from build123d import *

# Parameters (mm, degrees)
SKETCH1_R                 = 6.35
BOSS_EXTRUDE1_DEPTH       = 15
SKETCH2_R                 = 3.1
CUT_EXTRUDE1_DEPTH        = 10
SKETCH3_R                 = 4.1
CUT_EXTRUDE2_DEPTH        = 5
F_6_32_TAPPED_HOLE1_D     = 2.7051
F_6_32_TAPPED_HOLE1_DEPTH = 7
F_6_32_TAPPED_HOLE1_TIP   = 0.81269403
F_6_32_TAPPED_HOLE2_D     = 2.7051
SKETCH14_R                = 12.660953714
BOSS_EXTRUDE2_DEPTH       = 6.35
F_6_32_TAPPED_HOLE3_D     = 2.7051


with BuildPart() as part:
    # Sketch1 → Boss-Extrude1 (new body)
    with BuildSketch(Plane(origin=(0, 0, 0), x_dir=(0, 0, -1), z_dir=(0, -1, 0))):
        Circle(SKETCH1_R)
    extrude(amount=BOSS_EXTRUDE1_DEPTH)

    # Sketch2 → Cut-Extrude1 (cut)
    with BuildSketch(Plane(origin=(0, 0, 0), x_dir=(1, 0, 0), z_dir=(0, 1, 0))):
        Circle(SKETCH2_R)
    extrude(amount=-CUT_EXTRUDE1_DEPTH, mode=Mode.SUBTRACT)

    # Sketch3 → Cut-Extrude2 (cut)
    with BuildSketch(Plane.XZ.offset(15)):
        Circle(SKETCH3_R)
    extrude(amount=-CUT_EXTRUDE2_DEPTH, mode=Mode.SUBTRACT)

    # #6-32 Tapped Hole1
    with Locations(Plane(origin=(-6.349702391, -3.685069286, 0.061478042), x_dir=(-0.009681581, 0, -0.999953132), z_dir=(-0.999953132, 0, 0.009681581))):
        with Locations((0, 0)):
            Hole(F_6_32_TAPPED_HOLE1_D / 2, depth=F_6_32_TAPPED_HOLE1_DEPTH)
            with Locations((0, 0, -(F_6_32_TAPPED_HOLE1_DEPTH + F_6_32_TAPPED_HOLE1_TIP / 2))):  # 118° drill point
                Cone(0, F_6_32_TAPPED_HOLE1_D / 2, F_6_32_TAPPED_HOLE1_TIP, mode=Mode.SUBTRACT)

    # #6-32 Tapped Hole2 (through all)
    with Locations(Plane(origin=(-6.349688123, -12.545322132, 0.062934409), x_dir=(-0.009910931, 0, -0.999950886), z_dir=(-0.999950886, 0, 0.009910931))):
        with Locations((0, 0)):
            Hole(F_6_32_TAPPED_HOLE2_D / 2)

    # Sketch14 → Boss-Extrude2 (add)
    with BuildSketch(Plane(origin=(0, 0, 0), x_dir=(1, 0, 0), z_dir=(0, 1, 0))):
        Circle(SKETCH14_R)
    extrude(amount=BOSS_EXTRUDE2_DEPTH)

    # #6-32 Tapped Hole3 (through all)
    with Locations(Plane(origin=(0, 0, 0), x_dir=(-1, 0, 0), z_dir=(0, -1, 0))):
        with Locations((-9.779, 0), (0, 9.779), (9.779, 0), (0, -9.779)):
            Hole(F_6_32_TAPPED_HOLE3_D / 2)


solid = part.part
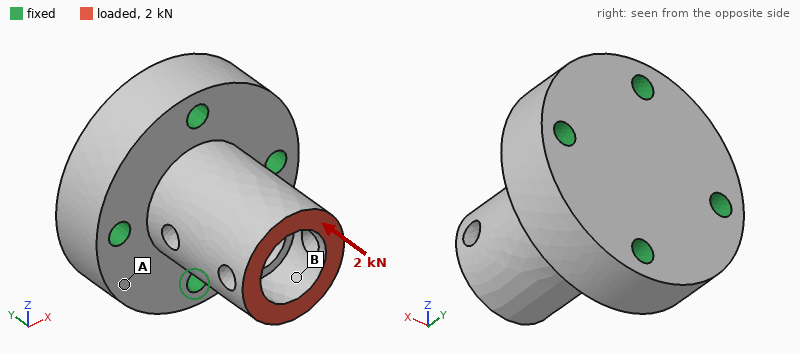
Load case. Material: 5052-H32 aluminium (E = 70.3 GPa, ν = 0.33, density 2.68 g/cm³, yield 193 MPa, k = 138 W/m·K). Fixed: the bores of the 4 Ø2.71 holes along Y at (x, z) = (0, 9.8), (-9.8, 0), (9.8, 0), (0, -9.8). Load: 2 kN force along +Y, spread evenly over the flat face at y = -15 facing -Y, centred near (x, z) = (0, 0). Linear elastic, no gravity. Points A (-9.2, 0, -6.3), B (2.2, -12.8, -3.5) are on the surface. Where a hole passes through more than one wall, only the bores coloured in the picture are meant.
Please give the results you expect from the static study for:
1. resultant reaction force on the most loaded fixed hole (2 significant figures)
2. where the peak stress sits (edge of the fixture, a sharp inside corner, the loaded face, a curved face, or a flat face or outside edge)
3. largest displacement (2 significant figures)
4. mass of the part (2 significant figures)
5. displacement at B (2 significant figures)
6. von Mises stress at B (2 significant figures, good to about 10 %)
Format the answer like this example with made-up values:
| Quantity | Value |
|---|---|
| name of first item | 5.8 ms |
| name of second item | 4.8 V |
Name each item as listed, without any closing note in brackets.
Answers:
| Quantity | Value |
|---|---|
| resultant reaction force on the most loaded fixed hole | 520 N |
| where the peak stress sits | a curved face |
| largest displacement | 11 µm |
| mass of the part | 12 g |
| displacement at B | 6.4 µm |
| von Mises stress at B | 31 MPa |
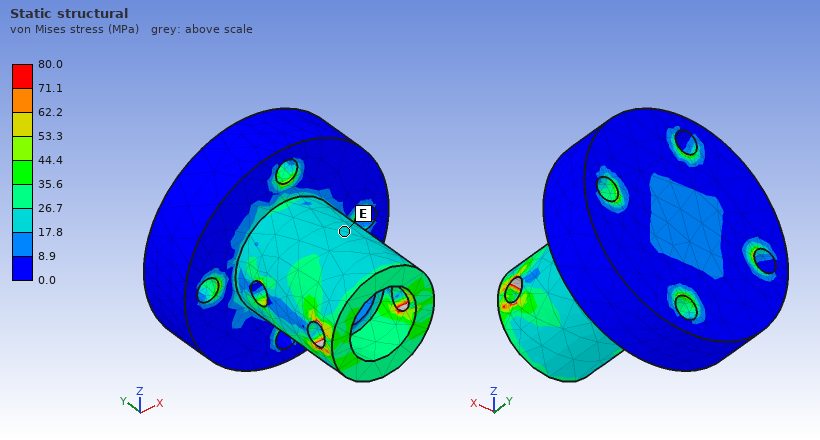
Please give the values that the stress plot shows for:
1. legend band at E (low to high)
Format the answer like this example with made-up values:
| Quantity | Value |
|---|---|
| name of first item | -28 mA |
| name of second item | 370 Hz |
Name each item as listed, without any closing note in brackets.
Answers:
| Quantity | Value |
|---|---|
| legend band at E | 17.8 to 26.7 MPa |
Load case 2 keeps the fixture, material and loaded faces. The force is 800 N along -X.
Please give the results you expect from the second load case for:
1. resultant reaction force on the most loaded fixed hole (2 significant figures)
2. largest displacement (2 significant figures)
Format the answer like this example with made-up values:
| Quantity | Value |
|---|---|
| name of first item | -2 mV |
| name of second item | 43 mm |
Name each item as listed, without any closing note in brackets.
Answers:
| Quantity | Value |
|---|---|
| resultant reaction force on the most loaded fixed hole | 790 N |
| largest displacement | 36 µm |
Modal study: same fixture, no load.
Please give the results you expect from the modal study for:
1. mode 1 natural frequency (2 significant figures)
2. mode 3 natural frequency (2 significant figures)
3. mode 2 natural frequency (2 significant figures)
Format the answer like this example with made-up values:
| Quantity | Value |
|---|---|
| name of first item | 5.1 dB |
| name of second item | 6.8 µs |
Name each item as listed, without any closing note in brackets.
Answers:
| Quantity | Value |
|---|---|
| mode 1 natural frequency | 26 kHz |
| mode 3 natural frequency | 48 kHz |
| mode 2 natural frequency | 26 kHz |
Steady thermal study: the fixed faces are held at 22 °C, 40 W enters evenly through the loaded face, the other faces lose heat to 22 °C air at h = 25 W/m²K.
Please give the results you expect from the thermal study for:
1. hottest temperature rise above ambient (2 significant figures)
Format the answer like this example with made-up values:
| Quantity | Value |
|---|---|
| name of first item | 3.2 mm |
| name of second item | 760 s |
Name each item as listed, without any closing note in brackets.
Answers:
| Quantity | Value |
|---|---|
| hottest temperature rise above ambient | 67 K |
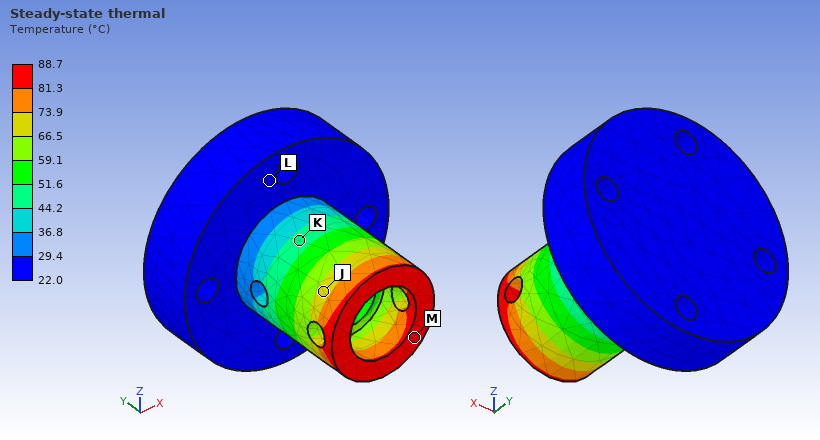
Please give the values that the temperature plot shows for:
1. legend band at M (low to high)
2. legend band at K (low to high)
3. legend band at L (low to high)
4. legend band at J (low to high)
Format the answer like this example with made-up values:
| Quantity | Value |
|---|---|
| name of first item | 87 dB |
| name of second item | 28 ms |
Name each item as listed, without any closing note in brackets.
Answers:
| Quantity | Value |
|---|---|
| legend band at M | 81.3 to 88.7 °C |
| legend band at K | 44.2 to 51.6 °C |
| legend band at L | 22.0 to 29.4 °C |
| legend band at J | 66.5 to 73.9 °C |
